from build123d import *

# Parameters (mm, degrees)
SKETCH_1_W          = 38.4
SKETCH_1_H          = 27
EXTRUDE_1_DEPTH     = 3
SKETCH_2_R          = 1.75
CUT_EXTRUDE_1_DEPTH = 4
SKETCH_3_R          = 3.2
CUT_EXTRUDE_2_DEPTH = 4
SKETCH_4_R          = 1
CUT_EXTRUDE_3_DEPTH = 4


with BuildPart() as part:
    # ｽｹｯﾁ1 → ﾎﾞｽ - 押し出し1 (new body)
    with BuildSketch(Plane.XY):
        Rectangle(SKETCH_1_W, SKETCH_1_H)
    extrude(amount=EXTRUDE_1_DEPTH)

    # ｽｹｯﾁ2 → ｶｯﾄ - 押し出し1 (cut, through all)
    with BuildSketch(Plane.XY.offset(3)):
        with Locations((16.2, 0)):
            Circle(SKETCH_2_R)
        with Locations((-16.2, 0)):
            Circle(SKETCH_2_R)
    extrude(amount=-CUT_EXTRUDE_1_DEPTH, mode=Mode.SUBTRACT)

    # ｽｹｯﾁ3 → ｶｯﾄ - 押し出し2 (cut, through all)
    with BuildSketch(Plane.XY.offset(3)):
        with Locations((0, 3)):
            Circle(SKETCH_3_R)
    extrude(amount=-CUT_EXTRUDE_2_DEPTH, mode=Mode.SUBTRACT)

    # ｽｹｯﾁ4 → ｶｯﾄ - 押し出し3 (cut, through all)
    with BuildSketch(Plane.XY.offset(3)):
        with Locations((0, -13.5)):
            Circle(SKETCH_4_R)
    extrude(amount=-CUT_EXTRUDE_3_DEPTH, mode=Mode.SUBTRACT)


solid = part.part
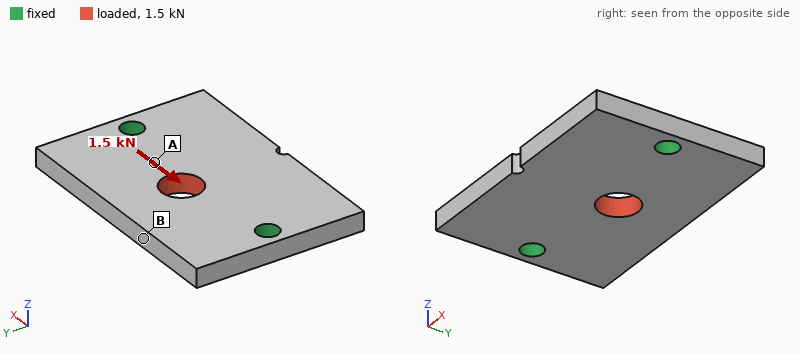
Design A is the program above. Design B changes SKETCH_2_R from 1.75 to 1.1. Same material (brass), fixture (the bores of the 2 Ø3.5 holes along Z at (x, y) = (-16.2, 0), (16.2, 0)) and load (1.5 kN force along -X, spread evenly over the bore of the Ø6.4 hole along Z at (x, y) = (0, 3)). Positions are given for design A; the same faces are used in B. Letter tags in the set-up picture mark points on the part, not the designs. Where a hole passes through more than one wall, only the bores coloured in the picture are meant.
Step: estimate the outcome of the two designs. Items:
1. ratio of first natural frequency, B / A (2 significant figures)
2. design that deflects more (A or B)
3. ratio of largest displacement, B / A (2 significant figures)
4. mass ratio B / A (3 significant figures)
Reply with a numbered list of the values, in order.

1. 0.86
2. B
3. 1.1
4. 1.01
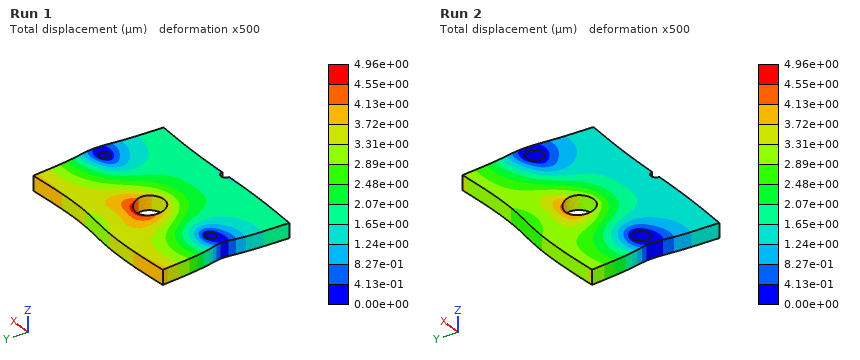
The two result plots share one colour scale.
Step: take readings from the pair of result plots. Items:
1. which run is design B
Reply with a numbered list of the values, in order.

1. Run 1
